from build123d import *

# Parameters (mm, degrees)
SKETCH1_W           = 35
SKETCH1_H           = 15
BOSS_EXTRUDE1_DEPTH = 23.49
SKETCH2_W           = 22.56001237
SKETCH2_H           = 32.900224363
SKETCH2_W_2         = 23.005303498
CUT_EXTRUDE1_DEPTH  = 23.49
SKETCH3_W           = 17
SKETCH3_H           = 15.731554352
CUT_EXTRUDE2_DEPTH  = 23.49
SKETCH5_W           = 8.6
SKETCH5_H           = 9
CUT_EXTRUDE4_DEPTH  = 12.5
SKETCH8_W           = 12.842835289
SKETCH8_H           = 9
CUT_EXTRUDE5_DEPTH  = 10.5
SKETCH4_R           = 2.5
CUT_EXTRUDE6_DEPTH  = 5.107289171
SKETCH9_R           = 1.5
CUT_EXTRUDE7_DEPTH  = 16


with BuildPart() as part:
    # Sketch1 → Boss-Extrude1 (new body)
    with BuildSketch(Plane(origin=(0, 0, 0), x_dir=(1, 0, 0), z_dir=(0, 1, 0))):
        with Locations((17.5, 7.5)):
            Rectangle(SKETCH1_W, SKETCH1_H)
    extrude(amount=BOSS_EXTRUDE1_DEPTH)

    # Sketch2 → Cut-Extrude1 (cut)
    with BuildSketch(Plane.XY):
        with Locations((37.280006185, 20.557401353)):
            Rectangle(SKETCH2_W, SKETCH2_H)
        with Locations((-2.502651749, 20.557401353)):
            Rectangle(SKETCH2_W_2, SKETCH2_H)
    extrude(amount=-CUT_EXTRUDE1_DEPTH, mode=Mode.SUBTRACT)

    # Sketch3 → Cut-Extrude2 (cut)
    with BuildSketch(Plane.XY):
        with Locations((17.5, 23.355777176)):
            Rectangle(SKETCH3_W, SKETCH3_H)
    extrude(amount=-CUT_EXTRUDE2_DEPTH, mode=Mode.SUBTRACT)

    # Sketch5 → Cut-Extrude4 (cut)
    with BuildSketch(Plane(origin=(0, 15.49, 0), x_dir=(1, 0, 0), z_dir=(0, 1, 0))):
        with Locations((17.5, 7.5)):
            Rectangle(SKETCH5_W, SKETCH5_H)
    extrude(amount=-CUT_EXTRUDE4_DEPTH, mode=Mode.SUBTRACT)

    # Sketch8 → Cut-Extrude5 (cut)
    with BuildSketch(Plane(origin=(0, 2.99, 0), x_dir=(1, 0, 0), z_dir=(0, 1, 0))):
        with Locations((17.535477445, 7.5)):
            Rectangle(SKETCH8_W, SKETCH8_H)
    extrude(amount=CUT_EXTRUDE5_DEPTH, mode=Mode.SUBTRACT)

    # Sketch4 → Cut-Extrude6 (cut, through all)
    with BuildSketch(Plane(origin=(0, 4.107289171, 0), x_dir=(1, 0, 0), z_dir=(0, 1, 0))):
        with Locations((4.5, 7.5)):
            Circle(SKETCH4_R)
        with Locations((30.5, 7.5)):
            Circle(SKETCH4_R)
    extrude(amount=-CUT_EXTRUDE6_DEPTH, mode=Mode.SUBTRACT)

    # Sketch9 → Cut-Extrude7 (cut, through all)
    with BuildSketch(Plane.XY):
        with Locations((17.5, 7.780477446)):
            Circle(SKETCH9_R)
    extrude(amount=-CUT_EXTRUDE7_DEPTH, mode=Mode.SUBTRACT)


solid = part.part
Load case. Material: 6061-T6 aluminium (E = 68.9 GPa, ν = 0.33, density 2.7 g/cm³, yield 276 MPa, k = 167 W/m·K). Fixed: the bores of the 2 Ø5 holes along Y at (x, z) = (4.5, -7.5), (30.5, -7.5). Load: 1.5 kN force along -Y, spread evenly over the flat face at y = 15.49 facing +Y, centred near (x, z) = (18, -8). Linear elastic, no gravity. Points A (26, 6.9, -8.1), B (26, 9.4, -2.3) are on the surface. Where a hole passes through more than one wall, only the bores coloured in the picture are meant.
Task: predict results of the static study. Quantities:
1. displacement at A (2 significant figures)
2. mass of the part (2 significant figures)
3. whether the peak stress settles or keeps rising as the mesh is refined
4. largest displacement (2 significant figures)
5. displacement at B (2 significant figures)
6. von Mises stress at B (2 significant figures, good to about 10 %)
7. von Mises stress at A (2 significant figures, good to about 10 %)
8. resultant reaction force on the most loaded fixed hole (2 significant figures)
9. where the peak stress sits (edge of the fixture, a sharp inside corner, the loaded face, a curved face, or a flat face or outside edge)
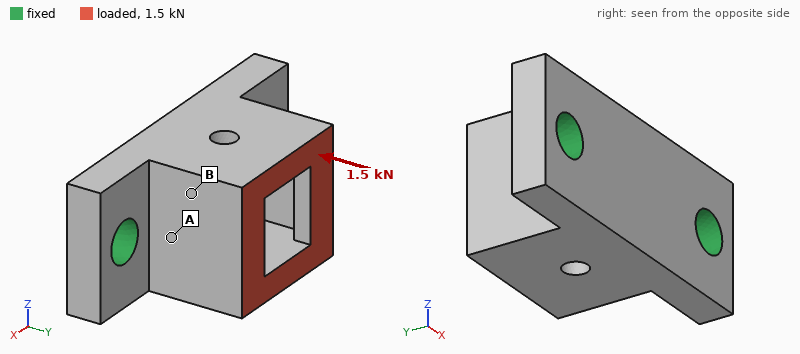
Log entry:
5.5 µm
9.4 g
keeps rising
11 µm
6.5 µm
12 MPa
31 MPa
760 N
edge of the fixture
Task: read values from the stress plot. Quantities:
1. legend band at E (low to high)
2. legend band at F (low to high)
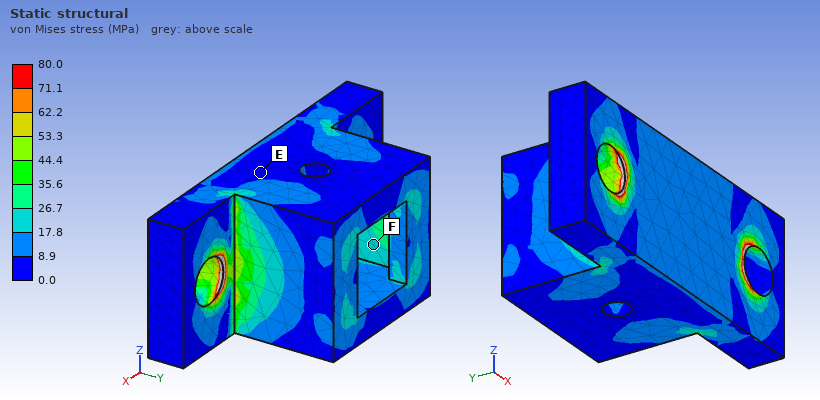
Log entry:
0.0 to 8.9 MPa
17.8 to 26.7 MPa
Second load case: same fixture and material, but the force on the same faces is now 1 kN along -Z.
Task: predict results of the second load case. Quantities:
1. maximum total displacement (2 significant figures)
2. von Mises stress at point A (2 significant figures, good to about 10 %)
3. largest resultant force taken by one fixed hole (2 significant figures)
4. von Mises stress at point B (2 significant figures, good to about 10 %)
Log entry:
62 µm
44 MPa
500 N
26 MPa
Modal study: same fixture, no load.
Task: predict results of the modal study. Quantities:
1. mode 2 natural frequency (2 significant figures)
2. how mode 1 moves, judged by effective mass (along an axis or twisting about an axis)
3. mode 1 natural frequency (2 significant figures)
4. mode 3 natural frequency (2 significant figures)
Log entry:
28 kHz
along Z
14 kHz
29 kHz
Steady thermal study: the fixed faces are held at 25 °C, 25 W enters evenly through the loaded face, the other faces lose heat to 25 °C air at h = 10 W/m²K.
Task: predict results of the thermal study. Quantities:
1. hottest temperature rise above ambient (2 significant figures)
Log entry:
22 K
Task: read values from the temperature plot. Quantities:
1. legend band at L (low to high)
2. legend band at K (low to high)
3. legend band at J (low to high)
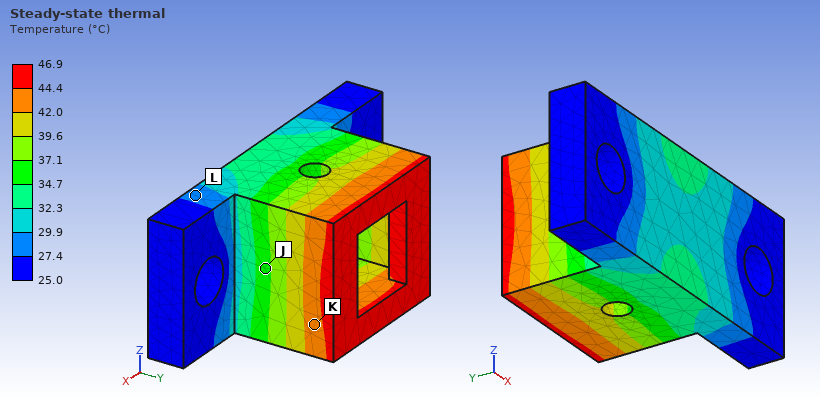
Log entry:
27.4 to 29.9 °C
42.0 to 44.4 °C
34.7 to 37.1 °C
